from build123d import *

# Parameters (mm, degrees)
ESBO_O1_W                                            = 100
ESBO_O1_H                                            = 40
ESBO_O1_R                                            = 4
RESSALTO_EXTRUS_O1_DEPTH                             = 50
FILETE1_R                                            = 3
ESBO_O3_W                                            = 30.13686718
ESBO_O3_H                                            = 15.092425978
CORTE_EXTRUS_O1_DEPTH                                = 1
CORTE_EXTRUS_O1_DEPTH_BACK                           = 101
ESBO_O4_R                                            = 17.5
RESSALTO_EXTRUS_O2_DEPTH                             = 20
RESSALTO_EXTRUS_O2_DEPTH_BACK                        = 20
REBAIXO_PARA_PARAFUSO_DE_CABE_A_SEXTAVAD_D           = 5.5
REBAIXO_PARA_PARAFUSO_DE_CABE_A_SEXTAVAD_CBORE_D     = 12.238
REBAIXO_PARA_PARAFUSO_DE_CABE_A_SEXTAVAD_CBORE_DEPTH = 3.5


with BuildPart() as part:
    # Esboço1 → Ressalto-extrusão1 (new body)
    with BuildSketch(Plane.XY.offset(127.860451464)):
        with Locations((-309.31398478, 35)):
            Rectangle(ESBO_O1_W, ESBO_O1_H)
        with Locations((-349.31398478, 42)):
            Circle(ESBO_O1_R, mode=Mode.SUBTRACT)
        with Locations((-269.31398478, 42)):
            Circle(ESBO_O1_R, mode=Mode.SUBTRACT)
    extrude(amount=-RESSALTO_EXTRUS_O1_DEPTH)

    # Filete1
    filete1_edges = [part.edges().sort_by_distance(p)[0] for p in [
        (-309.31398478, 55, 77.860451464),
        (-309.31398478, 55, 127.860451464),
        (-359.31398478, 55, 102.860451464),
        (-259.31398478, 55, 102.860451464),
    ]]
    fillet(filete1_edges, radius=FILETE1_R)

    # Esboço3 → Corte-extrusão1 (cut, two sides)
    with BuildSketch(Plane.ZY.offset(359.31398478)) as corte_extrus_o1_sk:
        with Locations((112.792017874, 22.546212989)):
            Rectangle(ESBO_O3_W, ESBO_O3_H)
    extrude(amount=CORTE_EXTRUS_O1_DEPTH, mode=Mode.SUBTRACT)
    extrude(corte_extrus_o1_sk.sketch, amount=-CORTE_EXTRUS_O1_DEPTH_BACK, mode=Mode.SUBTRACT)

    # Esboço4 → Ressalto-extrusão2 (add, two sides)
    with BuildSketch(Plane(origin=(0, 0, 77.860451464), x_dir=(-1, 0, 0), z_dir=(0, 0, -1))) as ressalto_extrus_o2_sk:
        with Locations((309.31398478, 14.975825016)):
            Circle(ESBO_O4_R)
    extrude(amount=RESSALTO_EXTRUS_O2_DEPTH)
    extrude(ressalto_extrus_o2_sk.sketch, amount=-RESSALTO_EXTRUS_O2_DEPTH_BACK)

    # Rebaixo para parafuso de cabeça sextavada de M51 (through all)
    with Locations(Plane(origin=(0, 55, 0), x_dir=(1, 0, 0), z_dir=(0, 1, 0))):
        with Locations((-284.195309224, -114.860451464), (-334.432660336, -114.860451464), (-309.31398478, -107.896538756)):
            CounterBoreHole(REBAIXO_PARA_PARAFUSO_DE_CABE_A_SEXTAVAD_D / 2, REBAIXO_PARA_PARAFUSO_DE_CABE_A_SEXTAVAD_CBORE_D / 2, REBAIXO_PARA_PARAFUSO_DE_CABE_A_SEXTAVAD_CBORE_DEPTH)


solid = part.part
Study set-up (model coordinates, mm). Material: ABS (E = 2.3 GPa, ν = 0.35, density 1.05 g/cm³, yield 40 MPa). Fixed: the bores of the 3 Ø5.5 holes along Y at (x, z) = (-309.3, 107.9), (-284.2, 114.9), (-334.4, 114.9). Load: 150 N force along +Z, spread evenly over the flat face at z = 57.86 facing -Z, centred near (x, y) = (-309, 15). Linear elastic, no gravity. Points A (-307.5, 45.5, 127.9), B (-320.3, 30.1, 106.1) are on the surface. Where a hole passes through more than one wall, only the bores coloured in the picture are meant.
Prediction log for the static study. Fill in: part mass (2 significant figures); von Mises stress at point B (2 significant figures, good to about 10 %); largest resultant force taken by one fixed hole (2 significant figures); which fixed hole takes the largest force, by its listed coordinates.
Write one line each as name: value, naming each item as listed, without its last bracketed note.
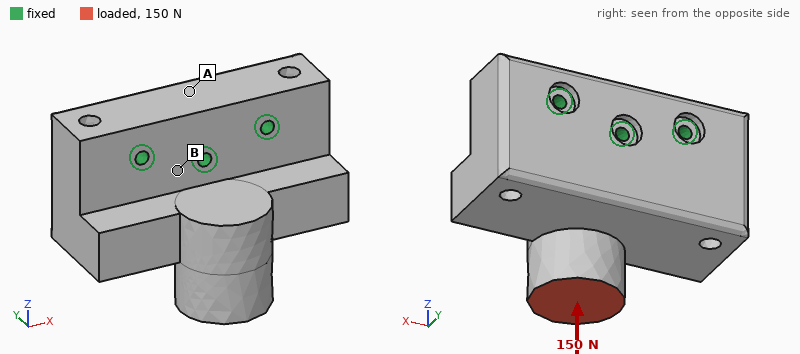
part mass: 180 g
von Mises stress at point B: 0.38 MPa
largest resultant force taken by one fixed hole: 81 N
which fixed hole takes the largest force, by its listed coordinates: (-309.3, 107.9)
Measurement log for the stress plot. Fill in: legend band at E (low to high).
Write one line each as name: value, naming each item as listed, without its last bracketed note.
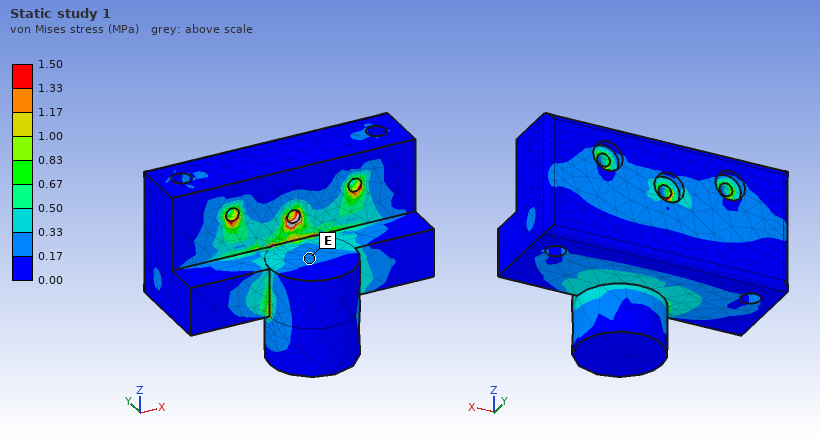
legend band at E: 0.17 to 0.33 MPa
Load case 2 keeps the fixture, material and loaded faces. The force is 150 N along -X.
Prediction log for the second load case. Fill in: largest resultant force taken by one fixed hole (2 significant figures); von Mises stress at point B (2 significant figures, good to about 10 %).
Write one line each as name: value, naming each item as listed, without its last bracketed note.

largest resultant force taken by one fixed hole: 160 N
von Mises stress at point B: 0.32 MPa
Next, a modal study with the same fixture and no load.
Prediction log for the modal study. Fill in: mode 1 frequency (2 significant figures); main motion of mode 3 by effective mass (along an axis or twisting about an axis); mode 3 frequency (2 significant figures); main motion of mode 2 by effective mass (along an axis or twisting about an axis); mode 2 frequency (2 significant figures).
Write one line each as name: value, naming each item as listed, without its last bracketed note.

mode 1 frequency: 1300 Hz
main motion of mode 3 by effective mass: along X
mode 3 frequency: 2600 Hz
main motion of mode 2 by effective mass: along X
mode 2 frequency: 2000 Hz
